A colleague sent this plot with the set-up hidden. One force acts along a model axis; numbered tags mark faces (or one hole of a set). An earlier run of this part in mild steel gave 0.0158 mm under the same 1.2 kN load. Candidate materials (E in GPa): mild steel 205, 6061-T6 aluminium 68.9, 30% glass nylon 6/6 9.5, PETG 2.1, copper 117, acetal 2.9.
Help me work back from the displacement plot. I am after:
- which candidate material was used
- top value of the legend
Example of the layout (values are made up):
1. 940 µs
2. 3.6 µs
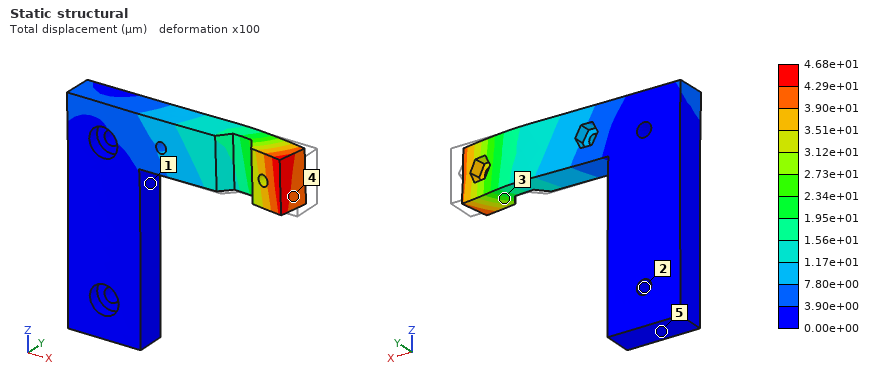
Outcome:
1. 6061-T6 aluminium
2. 4.68e+01 µm
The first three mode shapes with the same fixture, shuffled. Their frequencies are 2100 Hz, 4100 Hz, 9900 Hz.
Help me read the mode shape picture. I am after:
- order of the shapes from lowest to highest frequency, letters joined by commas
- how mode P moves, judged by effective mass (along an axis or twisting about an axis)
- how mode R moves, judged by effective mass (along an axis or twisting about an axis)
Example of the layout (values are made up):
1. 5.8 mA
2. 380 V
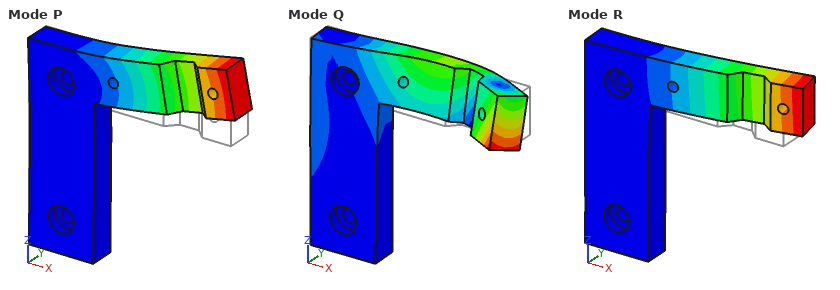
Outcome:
1. R, P, Q
2. along Z
3. along Y
